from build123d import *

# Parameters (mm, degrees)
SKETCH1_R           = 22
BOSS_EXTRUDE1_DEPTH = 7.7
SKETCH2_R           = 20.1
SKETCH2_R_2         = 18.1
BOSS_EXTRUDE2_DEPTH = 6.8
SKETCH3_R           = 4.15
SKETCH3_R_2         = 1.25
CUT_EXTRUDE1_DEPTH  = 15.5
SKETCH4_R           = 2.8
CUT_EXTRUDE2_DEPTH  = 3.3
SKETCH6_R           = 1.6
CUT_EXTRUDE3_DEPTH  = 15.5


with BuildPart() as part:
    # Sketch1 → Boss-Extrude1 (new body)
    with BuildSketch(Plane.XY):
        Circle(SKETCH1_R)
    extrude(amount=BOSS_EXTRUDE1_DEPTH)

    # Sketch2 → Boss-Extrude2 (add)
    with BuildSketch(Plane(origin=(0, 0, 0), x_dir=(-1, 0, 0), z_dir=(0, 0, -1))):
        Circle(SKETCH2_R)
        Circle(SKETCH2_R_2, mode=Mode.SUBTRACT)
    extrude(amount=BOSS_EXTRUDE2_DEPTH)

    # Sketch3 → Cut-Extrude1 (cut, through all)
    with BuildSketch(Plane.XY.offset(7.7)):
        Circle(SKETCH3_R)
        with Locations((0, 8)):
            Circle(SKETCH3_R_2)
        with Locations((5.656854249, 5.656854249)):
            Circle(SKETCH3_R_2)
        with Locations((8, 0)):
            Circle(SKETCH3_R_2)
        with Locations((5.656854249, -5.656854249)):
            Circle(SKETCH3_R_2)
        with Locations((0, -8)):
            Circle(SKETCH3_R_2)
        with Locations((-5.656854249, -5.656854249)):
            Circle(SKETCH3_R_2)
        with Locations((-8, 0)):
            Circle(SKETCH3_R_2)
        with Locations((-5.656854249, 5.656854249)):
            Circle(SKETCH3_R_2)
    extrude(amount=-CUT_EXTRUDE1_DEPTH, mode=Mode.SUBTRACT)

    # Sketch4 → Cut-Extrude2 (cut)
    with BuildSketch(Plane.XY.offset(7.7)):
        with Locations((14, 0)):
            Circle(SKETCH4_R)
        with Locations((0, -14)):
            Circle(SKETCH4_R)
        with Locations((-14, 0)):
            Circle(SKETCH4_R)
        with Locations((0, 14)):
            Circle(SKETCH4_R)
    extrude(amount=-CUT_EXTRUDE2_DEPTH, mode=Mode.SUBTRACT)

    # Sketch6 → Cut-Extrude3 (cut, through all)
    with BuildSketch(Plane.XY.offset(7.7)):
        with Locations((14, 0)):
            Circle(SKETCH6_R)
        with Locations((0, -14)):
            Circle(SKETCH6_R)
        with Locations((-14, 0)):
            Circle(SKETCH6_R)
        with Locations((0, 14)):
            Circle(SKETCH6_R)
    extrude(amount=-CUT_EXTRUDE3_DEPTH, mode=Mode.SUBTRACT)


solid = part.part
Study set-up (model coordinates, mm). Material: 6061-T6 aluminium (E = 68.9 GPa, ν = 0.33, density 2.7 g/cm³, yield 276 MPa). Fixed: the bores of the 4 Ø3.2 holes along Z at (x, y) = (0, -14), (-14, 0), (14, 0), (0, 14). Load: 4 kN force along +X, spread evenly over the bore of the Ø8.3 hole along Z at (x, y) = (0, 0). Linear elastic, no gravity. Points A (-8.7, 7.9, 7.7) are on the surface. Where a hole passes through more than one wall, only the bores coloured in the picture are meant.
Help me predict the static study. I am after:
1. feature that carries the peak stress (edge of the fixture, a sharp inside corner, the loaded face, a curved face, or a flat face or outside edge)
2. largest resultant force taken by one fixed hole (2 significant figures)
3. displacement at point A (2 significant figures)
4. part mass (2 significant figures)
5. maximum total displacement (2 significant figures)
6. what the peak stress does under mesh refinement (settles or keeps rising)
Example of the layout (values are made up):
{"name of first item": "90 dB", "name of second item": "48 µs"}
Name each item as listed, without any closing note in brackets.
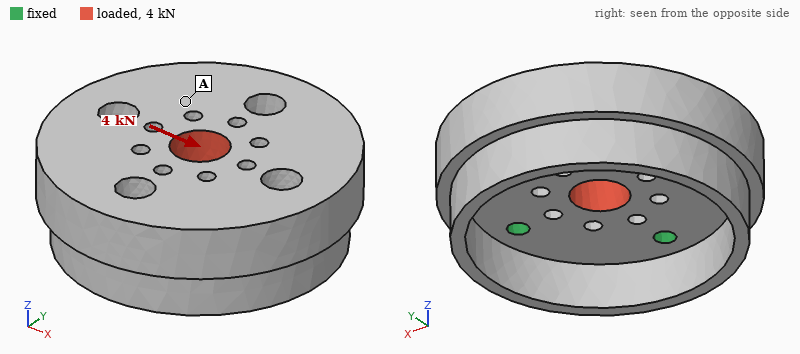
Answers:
{"feature that carries the peak stress": "edge of the fixture", "largest resultant force taken by one fixed hole": "1.2 kN", "displacement at point A": "2.3 µm", "part mass": "33 g", "maximum total displacement": "4.8 µm", "what the peak stress does under mesh refinement": "keeps rising"}
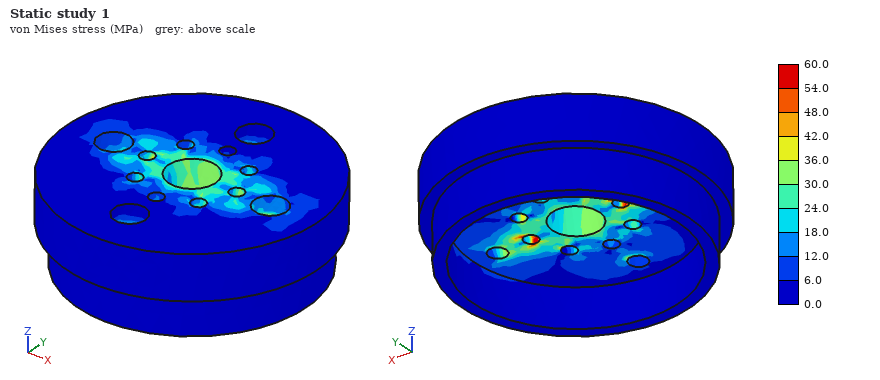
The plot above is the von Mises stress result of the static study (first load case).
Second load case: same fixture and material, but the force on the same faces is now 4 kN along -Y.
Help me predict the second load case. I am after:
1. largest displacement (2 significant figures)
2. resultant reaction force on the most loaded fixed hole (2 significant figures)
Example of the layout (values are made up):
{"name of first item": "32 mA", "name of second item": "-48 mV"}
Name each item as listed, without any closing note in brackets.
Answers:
{"largest displacement": "4.8 µm", "resultant reaction force on the most loaded fixed hole": "1.2 kN"}
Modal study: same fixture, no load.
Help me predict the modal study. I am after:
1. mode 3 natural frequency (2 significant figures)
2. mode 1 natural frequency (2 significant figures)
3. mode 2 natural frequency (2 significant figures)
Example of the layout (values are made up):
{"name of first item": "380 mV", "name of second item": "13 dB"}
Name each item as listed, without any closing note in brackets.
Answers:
{"mode 3 natural frequency": "25 kHz", "mode 1 natural frequency": "20 kHz", "mode 2 natural frequency": "25 kHz"}
